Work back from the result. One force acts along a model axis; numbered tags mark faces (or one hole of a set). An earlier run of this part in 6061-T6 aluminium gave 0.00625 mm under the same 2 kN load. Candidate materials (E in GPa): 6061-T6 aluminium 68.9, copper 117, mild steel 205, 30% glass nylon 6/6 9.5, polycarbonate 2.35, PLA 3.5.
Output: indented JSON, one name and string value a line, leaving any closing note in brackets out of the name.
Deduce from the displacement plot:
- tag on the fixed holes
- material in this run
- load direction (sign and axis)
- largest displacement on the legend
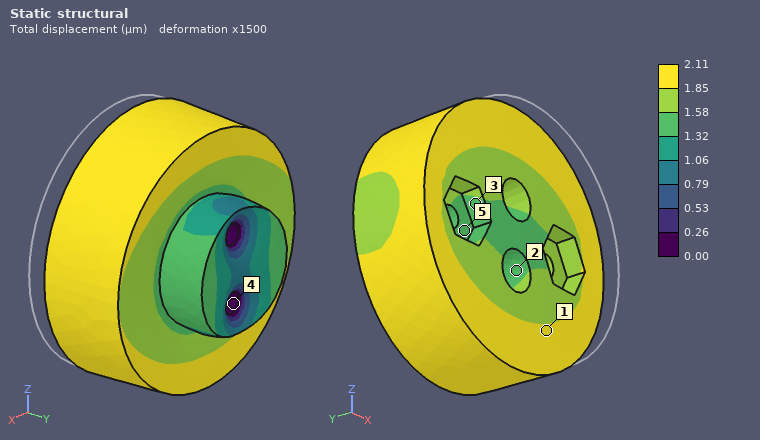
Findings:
{
  "tag on the fixed holes": "4",
  "material in this run": "mild steel",
  "load direction": "+Y",
  "largest displacement on the legend": "2.11 µm"
}
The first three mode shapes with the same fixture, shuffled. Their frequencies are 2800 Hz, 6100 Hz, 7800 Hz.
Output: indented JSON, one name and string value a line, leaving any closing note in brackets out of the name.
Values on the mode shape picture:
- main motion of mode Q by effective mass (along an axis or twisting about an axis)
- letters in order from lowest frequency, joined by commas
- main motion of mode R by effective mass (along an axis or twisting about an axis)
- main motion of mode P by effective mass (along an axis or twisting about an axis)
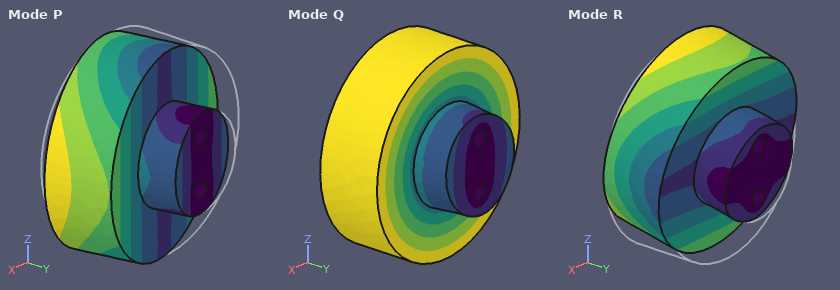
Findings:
{
  "main motion of mode Q by effective mass": "twisting about Y",
  "letters in order from lowest frequency, joined by commas": "P, R, Q",
  "main motion of mode R by effective mass": "along Z",
  "main motion of mode P by effective mass": "along X"
}
